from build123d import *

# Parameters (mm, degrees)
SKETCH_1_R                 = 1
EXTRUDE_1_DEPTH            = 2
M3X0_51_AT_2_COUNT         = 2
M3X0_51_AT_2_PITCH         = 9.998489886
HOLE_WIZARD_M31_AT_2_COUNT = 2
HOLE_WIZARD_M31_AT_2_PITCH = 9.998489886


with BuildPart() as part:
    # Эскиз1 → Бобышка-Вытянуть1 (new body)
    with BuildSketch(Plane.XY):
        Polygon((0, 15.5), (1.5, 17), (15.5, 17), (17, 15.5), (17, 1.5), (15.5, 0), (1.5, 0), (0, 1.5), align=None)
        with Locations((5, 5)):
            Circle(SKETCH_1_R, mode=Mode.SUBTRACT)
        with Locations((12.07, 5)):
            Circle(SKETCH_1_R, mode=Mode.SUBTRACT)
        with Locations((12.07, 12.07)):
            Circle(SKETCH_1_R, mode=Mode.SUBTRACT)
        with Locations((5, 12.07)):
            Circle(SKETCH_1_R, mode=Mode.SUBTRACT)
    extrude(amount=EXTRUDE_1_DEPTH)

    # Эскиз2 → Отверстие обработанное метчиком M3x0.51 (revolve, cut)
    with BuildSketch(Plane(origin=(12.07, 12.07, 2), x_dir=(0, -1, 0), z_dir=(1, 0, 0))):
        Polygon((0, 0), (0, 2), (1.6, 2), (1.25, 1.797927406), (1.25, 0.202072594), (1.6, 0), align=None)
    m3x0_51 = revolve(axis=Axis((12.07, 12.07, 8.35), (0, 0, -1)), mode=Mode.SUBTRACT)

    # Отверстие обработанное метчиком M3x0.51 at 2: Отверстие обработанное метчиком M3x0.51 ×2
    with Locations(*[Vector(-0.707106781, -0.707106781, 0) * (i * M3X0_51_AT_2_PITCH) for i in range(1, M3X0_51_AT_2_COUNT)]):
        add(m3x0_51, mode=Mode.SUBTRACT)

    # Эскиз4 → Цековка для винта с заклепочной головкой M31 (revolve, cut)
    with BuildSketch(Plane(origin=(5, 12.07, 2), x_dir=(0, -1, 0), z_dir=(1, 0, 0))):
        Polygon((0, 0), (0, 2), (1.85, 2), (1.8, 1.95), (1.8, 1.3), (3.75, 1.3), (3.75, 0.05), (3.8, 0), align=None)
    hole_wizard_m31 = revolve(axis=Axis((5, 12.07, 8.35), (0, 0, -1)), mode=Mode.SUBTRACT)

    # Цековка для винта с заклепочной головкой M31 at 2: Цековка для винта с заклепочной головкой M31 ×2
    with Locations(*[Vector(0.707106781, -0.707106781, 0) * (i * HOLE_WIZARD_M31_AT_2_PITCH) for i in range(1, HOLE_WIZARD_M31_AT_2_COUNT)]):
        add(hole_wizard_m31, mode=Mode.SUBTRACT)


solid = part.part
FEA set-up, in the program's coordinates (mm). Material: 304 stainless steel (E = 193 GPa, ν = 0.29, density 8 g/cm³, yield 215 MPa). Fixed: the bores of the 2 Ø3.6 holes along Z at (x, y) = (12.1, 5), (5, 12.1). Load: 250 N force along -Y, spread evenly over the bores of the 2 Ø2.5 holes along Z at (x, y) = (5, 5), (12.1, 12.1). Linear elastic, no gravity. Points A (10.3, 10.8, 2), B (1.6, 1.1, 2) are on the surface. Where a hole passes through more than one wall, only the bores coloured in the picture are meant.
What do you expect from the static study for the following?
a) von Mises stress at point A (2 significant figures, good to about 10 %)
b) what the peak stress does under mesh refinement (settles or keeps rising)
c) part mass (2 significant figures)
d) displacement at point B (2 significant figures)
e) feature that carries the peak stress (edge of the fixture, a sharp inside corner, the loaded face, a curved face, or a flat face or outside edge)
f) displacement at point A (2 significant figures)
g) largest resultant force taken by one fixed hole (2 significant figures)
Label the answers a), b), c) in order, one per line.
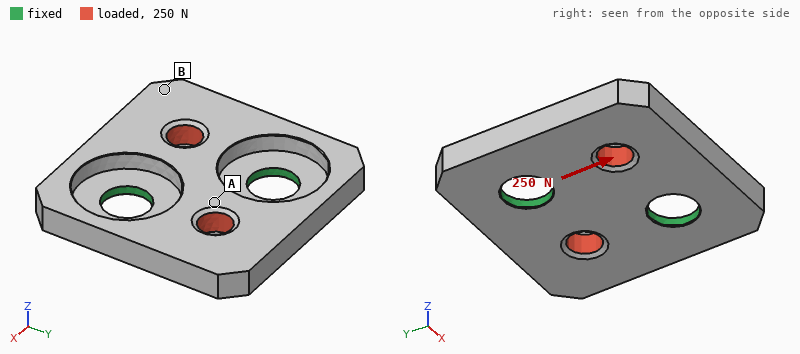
a) 14 MPa
b) keeps rising
c) 3.4 g
d) 3.8 µm
e) edge of the fixture
f) 1.2 µm
g) 130 N
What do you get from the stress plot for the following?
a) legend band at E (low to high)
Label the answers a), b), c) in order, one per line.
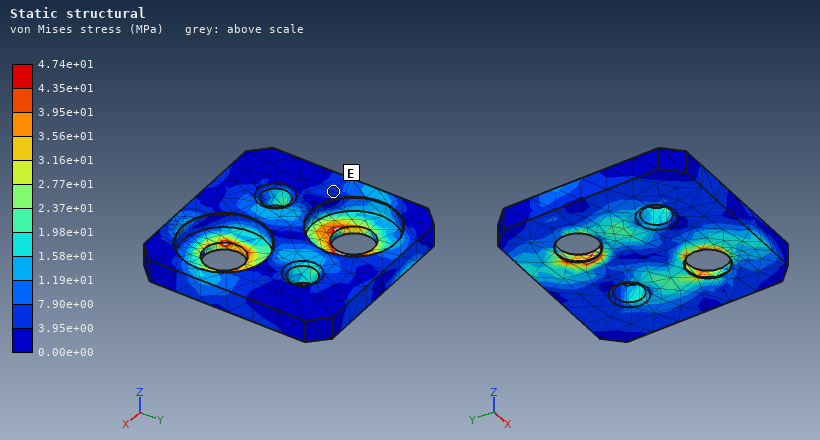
a) 3.95e+00 to 7.90e+00 MPa
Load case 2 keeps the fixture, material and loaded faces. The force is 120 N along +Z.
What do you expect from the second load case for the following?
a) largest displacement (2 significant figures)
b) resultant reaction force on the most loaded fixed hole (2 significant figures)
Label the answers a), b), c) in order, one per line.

a) 7.7 µm
b) 75 N
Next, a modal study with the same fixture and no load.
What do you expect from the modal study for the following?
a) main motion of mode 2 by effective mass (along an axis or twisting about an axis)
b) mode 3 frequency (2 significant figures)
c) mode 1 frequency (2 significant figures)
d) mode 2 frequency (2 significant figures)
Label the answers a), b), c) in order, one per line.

a) along Z
b) 33 kHz
c) 10 kHz
d) 15 kHz
